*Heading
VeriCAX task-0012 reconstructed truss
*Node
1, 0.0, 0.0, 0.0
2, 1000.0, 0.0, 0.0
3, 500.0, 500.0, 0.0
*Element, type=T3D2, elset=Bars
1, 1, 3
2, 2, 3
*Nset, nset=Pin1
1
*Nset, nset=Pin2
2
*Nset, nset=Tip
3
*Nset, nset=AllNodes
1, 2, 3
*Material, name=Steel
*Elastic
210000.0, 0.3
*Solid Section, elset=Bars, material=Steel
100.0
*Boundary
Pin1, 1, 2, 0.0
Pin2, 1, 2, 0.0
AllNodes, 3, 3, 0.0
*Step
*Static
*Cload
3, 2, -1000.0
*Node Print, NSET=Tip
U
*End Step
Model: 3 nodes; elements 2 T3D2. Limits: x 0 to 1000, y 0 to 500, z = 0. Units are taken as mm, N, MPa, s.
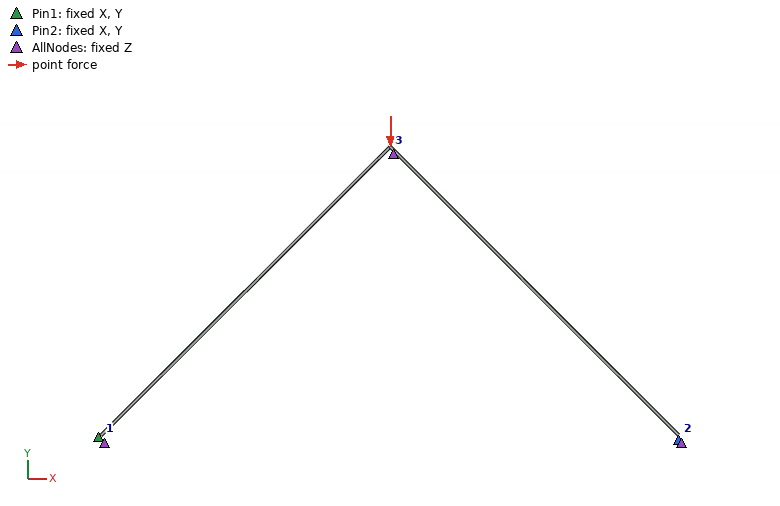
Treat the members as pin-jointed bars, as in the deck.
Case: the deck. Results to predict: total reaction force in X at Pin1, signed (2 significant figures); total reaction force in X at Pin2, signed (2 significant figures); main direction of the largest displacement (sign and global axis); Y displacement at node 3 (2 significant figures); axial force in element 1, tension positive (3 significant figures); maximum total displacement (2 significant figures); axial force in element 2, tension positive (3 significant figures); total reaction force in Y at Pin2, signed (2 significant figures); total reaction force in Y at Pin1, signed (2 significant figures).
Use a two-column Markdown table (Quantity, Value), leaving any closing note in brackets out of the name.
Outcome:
| Quantity | Value |
|---|---|
| total reaction force in X at Pin1, signed | 500 N |
| total reaction force in X at Pin2, signed | -500 N |
| main direction of the largest displacement | -Y |
| Y displacement at node 3 | -0.034 mm |
| axial force in element 1, tension positive | -707 N |
| maximum total displacement | 0.034 mm |
| axial force in element 2, tension positive | -707 N |
| total reaction force in Y at Pin2, signed | 500 N |
| total reaction force in Y at Pin1, signed | 500 N |
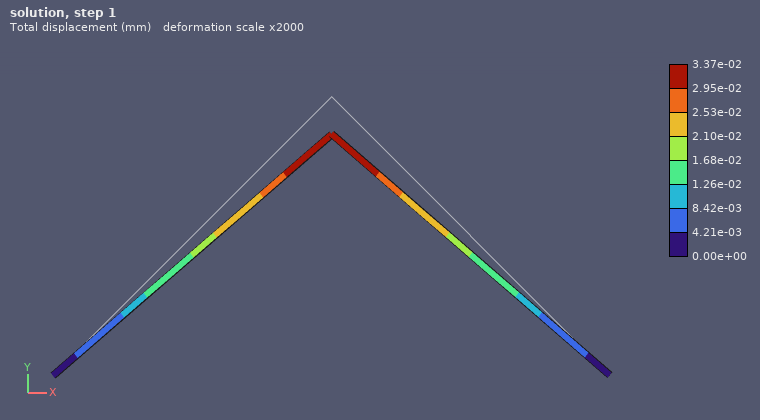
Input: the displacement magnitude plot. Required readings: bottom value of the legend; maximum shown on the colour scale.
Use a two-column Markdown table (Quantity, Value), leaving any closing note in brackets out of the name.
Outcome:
| Quantity | Value |
|---|---|
| bottom value of the legend | 0.00e+00 mm |
| maximum shown on the colour scale | 3.37e-02 mm |
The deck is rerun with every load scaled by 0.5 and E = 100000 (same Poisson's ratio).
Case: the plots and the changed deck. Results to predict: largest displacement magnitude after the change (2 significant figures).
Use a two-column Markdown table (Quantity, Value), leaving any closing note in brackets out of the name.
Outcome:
| Quantity | Value |
|---|---|
| largest displacement magnitude after the change | 0.035 mm |
